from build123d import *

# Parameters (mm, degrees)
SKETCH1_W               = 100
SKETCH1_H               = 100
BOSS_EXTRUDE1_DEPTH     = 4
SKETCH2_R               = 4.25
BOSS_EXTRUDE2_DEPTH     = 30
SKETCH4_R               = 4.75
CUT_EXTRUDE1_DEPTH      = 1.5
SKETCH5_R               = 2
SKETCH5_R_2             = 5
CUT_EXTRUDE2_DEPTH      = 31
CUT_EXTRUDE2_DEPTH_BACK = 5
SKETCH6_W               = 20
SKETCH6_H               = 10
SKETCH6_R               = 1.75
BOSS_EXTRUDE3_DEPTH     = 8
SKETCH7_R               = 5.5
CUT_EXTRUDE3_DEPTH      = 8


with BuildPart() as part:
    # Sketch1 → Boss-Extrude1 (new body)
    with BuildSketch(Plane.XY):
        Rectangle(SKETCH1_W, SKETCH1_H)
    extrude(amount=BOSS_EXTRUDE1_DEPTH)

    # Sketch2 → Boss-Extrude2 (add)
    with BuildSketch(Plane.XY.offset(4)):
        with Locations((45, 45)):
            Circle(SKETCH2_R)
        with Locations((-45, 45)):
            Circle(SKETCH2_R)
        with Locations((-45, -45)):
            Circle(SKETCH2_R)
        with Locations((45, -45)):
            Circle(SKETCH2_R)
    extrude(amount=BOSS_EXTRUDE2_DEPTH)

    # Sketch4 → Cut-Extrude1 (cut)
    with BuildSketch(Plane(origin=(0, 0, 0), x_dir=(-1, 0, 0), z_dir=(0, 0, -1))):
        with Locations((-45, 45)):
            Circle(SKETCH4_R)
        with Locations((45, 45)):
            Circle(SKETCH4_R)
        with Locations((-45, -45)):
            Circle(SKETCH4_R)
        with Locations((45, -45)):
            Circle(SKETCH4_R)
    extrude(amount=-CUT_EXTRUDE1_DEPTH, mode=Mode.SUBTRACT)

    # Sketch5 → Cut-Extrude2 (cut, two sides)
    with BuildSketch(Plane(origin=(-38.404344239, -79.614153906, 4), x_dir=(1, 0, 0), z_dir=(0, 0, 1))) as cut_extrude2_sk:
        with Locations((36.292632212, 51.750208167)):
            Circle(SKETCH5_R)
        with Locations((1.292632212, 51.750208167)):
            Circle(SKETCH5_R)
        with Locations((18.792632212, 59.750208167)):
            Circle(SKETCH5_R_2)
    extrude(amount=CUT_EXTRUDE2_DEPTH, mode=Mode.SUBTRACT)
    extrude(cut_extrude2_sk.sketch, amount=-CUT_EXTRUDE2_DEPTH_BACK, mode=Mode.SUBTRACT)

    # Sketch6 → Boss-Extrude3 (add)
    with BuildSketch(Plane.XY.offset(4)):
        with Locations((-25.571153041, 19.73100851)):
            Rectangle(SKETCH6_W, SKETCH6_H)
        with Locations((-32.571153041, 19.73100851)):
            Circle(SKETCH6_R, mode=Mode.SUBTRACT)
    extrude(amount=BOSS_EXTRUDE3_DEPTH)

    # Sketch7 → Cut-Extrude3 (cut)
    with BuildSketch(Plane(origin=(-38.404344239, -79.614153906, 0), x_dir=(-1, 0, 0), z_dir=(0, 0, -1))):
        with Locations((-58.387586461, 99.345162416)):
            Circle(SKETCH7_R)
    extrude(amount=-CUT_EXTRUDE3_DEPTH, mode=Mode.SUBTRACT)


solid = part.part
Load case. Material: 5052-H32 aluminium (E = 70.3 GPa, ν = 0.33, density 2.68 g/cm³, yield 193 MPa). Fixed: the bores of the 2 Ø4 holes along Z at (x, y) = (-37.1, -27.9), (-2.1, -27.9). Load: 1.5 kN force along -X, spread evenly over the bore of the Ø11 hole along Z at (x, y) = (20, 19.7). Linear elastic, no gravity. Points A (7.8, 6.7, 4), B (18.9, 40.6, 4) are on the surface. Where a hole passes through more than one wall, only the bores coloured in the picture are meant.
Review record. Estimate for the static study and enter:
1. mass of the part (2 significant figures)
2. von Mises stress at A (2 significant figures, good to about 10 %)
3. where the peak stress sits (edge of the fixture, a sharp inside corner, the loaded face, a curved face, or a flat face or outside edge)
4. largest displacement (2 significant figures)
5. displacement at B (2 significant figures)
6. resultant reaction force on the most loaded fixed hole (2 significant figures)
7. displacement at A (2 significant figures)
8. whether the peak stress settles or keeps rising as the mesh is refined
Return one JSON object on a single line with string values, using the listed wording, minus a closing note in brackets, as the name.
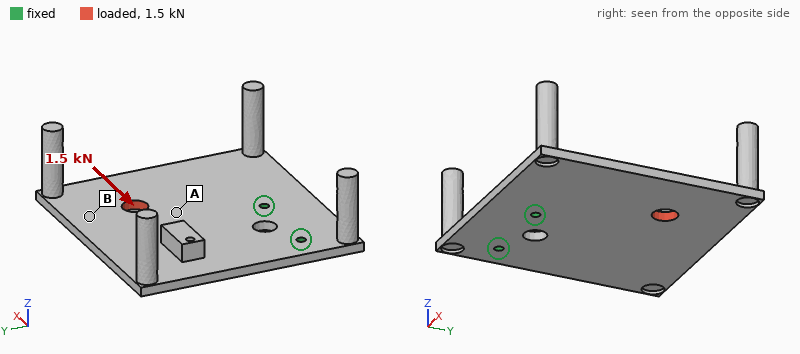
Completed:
{"mass of the part": "130 g", "von Mises stress at A": "11 MPa", "where the peak stress sits": "edge of the fixture", "largest displacement": "57 µm", "displacement at B": "46 µm", "resultant reaction force on the most loaded fixed hole": "2.1 kN", "displacement at A": "26 µm", "whether the peak stress settles or keeps rising as the mesh is refined": "keeps rising"}
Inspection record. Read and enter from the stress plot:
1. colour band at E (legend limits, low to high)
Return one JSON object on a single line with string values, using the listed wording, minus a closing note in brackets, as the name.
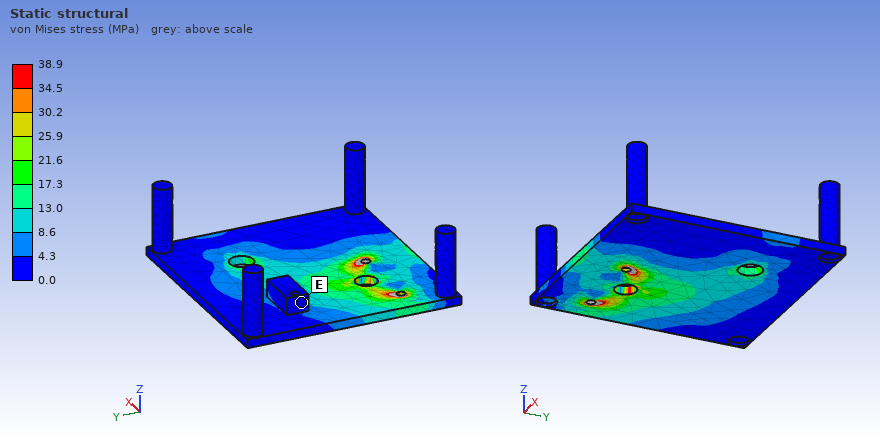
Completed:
{"colour band at E": "0.0 to 4.3 MPa"}
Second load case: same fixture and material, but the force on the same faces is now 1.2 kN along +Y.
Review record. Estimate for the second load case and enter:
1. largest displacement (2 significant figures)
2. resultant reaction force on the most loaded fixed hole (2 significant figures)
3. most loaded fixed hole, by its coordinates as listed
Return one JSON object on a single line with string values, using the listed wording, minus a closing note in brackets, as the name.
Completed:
{"largest displacement": "33 µm", "resultant reaction force on the most loaded fixed hole": "1.9 kN", "most loaded fixed hole, by its coordinates as listed": "(-2.1, -27.9)"}
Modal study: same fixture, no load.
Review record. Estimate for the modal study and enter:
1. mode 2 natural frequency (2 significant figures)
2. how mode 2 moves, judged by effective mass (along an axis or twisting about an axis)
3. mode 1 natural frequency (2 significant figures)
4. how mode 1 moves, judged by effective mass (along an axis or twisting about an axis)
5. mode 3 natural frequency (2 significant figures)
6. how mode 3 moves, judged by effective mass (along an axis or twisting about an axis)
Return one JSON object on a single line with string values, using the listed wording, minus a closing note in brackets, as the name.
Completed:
{"mode 2 natural frequency": "640 Hz", "how mode 2 moves, judged by effective mass": "twisting about Y", "mode 1 natural frequency": "380 Hz", "how mode 1 moves, judged by effective mass": "along Z", "mode 3 natural frequency": "1000 Hz", "how mode 3 moves, judged by effective mass": "along Z"}
